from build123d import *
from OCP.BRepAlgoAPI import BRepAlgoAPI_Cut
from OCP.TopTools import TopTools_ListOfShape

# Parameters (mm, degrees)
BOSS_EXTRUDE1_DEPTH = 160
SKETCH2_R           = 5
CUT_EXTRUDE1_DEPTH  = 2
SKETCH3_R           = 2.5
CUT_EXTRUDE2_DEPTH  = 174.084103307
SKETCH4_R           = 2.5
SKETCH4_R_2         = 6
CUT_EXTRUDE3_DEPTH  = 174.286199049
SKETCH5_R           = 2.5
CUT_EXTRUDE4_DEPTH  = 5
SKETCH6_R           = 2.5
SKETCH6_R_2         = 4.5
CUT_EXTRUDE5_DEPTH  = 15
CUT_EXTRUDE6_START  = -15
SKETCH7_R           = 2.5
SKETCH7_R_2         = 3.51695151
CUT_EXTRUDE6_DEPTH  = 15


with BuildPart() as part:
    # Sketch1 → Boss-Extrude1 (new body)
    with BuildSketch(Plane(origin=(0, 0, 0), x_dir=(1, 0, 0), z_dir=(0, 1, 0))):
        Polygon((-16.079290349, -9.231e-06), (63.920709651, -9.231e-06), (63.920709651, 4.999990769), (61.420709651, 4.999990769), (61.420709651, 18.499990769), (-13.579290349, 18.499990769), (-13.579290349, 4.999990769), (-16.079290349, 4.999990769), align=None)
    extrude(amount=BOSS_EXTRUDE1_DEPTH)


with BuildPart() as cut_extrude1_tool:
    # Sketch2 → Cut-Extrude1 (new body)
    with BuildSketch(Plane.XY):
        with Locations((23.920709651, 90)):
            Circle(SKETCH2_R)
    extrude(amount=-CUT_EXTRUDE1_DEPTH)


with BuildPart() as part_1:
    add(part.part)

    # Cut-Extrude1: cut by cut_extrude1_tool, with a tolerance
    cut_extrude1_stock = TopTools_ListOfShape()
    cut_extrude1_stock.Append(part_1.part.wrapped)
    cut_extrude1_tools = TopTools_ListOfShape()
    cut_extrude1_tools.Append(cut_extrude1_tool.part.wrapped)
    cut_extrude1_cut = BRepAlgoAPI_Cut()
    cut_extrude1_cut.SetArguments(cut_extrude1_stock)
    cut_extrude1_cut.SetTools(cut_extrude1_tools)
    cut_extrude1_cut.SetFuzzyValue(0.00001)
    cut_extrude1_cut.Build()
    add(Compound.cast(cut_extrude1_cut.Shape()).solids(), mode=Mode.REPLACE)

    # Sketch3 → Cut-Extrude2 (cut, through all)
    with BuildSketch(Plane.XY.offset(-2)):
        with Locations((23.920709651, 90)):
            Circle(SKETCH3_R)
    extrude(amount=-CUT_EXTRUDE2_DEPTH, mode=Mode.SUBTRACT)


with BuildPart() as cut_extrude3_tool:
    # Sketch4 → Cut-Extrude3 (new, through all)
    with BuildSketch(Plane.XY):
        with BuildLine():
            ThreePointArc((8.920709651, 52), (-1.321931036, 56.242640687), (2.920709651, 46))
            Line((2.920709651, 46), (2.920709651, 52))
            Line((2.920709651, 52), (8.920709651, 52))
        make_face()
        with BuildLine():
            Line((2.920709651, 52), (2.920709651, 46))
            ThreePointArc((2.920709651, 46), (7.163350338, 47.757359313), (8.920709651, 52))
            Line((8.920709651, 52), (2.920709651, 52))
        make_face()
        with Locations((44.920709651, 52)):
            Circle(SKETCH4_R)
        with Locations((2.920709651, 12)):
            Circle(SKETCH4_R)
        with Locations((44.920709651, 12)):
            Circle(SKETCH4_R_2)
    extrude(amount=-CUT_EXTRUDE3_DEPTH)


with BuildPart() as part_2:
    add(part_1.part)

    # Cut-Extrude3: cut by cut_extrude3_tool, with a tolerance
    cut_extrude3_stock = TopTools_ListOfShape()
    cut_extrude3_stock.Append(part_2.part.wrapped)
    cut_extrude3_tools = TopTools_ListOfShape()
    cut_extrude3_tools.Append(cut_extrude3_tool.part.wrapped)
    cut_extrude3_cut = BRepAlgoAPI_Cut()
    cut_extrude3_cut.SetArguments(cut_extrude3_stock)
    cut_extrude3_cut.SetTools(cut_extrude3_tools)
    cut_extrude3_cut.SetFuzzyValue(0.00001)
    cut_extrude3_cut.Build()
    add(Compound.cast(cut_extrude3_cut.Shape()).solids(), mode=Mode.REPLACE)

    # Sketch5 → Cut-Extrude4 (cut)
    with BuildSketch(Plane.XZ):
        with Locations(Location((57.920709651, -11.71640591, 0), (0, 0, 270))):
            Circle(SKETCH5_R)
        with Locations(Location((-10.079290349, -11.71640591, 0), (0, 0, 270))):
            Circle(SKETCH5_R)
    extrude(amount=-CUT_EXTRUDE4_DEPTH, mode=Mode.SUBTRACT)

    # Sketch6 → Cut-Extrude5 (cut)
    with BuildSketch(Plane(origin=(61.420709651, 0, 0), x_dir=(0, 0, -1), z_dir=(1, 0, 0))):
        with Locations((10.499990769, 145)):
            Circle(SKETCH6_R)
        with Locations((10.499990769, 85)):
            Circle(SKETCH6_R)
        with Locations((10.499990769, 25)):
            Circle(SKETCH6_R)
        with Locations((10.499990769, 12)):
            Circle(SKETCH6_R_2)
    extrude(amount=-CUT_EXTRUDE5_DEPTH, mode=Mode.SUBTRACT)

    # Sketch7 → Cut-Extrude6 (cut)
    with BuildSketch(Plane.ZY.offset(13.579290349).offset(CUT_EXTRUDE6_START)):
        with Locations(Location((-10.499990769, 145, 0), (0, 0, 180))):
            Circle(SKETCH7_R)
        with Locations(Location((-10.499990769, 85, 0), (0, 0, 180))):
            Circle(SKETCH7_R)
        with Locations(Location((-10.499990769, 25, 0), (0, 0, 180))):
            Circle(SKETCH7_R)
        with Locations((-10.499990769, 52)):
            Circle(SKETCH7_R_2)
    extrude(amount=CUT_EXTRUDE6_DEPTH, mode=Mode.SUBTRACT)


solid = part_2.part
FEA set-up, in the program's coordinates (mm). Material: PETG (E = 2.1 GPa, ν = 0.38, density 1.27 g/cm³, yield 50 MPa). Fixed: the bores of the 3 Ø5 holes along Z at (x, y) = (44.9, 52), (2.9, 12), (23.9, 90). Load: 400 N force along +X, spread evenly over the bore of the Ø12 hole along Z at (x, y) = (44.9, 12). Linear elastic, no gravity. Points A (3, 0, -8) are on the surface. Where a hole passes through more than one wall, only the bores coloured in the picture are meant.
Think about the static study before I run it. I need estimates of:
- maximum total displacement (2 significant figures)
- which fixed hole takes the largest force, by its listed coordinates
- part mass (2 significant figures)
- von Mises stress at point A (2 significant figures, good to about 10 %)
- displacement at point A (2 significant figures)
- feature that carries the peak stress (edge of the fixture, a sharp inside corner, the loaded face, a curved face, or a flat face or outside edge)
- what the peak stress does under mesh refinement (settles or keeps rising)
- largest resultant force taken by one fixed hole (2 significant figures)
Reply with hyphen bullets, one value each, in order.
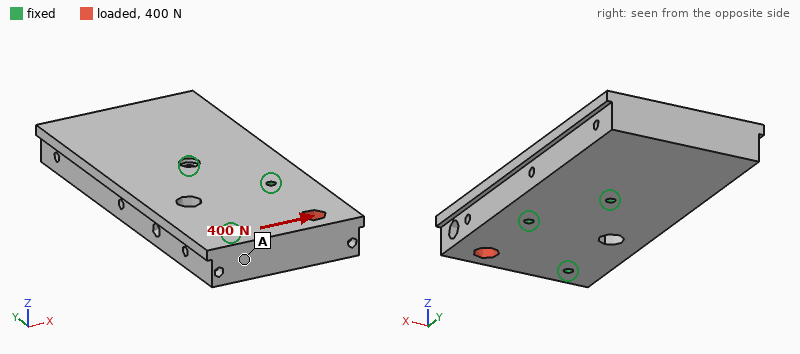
- 22 µm
- (2.9, 12)
- 280 g
- 0.29 MPa
- 3.9 µm
- edge of the fixture
- keeps rising
- 320 N
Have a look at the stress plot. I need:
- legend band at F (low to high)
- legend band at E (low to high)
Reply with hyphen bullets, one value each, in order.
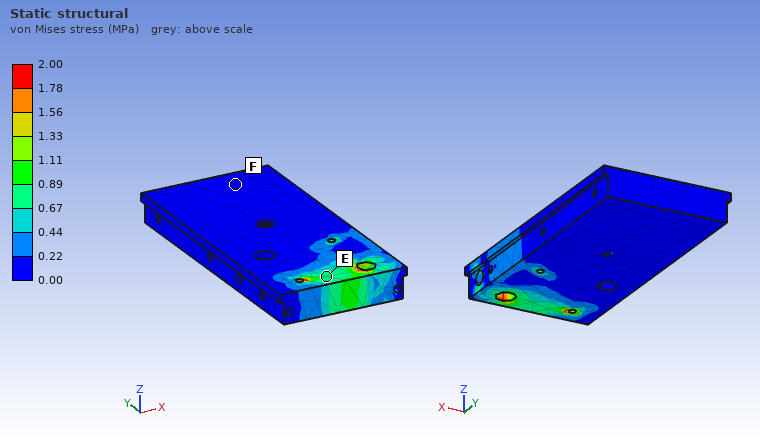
- 0.00 to 0.22 MPa
- 0.67 to 0.89 MPa
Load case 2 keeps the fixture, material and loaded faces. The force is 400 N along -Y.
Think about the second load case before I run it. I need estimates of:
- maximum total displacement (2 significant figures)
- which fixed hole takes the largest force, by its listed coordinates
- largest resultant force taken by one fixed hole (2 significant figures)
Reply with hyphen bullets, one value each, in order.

- 24 µm
- (44.9, 52)
- 270 N
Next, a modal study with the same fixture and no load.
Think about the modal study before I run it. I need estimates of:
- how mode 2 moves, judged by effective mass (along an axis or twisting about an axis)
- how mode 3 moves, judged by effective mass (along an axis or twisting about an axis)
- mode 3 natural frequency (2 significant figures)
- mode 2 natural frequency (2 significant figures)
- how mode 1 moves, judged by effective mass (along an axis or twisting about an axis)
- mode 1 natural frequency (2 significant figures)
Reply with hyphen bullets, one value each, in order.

- twisting about Y
- along X
- 1200 Hz
- 950 Hz
- along Z
- 590 Hz
